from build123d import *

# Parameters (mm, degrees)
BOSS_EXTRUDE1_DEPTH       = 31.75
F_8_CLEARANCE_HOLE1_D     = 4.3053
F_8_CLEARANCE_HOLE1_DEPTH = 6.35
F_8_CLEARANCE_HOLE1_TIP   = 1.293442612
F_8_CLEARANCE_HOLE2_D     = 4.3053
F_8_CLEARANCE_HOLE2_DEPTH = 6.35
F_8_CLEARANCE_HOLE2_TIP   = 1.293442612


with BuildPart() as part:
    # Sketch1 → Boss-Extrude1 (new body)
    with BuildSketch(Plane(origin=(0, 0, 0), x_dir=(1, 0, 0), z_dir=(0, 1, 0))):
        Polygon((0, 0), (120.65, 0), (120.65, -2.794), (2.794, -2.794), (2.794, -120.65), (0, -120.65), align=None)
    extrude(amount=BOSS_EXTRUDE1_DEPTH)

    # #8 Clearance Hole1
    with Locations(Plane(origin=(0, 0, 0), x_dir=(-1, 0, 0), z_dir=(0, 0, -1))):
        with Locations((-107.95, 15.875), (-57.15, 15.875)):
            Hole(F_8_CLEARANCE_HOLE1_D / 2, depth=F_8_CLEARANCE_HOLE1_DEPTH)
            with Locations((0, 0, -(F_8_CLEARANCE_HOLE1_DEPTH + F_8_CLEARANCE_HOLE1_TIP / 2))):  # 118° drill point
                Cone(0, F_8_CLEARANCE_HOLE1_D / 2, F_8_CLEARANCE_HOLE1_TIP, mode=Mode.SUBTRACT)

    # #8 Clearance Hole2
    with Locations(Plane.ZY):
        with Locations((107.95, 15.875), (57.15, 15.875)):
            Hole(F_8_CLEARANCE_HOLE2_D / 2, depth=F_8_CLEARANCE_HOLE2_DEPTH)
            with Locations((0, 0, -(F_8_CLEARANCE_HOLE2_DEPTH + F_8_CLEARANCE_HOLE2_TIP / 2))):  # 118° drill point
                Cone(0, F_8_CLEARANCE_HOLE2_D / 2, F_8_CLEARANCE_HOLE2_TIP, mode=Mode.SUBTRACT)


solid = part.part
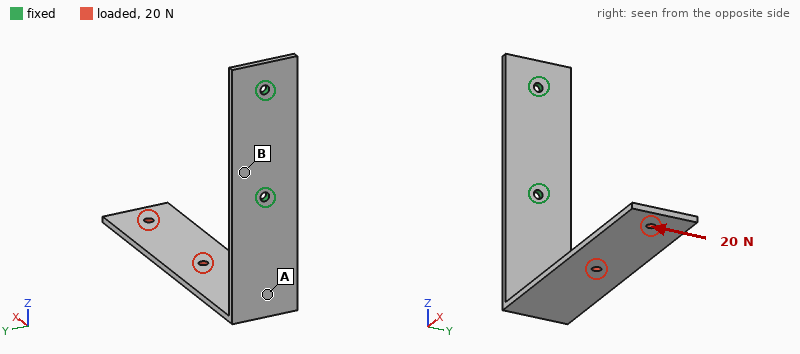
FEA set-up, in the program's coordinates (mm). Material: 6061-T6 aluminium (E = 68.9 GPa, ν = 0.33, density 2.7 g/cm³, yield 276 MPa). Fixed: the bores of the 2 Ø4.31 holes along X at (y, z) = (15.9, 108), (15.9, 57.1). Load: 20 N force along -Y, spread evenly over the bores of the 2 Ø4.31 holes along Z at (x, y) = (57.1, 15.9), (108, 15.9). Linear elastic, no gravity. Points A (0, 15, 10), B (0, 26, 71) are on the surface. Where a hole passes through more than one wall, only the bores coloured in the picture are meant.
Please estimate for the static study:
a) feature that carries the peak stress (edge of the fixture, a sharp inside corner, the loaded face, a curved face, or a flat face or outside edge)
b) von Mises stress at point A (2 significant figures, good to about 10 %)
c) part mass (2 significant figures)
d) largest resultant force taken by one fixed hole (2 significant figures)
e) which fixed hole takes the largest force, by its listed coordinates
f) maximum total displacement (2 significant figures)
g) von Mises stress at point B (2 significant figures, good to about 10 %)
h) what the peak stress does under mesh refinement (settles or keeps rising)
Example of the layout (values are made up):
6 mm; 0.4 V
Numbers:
edge of the fixture; 29 MPa; 57 g; 39 N; (15.9, 57.1); 1.8 mm; 6.6 MPa; keeps rising
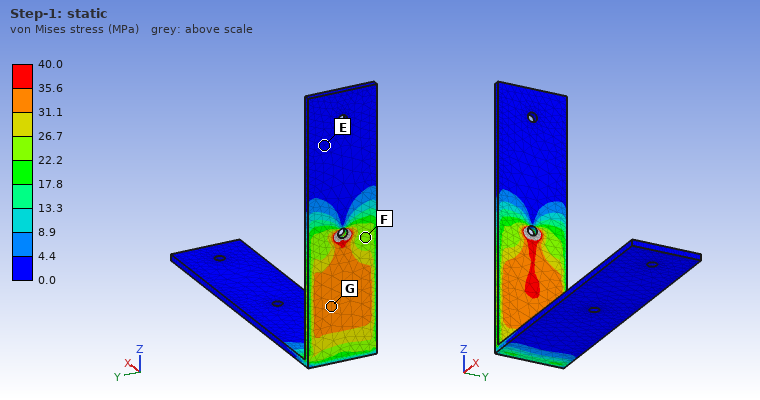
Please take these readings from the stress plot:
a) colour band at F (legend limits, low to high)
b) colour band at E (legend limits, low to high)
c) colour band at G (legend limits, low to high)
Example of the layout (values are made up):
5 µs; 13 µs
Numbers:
22.2 to 26.7 MPa; 0.0 to 4.4 MPa; 31.1 to 35.6 MPa
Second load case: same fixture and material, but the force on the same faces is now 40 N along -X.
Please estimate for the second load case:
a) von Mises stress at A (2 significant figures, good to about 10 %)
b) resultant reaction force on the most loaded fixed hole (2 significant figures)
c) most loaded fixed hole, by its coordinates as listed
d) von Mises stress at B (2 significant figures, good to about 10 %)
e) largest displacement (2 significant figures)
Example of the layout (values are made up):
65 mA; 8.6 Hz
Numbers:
8.3 MPa; 47 N; (15.9, 57.1); 5.7 MPa; 1.9 mm
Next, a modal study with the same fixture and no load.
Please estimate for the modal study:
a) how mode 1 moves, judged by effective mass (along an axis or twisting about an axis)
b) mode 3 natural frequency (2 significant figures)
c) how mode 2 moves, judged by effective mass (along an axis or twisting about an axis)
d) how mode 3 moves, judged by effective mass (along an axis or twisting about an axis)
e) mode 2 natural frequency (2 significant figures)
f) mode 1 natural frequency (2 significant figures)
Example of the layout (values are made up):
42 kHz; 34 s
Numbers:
along Z; 340 Hz; along Y; along X; 140 Hz; 92 Hz
